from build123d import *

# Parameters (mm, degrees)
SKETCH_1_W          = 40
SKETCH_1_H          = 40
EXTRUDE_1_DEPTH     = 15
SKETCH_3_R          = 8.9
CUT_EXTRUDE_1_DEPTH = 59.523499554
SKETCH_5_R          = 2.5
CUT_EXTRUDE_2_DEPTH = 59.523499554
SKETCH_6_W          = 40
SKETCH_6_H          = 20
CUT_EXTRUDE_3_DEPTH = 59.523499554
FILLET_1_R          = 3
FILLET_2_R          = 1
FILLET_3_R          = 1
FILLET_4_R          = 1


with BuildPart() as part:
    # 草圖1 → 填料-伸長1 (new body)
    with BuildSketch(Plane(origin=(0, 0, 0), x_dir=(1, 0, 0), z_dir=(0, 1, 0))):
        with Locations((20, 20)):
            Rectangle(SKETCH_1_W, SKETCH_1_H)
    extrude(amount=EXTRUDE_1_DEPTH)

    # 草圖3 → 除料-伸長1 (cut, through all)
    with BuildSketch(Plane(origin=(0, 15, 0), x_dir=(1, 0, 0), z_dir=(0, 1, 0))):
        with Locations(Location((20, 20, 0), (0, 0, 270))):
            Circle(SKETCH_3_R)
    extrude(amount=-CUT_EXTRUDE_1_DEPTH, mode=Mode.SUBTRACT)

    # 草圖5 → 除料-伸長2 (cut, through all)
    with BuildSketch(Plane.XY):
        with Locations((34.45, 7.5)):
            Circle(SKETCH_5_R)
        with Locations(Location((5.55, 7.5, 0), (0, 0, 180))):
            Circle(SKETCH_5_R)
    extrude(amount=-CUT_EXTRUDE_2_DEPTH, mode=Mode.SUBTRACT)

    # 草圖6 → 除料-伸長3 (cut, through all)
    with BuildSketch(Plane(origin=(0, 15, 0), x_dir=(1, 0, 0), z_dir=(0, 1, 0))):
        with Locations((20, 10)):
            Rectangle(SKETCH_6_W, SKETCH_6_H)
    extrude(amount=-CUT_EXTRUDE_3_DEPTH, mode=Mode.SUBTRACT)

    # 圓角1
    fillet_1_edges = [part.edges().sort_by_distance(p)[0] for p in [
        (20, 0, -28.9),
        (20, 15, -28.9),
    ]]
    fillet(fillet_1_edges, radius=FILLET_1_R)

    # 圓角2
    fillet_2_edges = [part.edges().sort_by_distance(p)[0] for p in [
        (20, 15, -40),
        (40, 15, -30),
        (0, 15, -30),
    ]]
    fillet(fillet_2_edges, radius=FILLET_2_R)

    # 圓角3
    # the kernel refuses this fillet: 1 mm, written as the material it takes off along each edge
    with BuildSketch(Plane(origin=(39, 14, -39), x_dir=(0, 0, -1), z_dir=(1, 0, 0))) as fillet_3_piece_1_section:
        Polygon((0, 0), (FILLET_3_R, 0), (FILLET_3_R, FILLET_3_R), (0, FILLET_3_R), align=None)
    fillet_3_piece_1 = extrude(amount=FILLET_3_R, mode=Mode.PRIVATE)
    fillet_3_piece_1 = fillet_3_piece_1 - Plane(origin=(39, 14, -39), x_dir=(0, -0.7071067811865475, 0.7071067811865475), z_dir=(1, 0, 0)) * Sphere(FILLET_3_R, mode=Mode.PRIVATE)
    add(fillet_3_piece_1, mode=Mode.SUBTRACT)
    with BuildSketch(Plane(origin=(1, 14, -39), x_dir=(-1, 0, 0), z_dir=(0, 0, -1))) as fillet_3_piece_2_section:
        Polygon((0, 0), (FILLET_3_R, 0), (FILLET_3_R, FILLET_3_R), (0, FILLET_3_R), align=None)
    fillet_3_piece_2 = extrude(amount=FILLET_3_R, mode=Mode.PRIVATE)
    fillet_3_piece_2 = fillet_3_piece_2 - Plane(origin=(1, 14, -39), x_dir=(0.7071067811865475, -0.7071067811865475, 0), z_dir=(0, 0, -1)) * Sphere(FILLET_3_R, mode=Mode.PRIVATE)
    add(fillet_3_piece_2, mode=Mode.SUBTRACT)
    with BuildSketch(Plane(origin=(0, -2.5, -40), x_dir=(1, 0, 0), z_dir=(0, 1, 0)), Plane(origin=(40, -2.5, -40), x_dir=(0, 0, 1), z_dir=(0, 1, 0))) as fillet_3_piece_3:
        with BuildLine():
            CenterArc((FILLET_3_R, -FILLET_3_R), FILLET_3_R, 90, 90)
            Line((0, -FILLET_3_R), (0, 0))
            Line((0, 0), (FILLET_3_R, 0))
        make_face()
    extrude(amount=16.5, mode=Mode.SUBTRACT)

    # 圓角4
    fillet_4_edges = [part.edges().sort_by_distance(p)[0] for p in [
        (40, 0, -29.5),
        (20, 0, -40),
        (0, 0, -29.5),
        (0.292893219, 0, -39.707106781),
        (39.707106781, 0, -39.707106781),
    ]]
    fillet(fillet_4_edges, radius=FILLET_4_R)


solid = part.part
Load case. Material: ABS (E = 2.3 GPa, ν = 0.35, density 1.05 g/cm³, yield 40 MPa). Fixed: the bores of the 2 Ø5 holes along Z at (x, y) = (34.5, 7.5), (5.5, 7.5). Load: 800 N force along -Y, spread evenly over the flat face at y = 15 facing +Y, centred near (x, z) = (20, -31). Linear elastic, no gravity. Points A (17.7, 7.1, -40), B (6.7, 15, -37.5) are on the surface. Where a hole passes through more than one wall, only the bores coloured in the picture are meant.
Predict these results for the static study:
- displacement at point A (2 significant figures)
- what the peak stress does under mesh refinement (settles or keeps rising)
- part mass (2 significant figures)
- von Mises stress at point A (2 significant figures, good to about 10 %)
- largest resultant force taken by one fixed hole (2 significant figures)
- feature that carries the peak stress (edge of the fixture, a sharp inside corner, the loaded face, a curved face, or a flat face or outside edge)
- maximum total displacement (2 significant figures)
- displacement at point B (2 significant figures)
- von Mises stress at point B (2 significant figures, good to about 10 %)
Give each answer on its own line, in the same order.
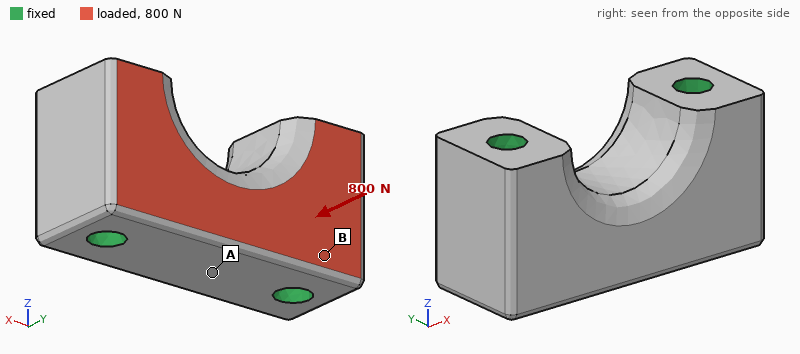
15 µm
keeps rising
9.7 g
0.77 MPa
400 N
edge of the fixture
17 µm
5.7 µm
2.0 MPa
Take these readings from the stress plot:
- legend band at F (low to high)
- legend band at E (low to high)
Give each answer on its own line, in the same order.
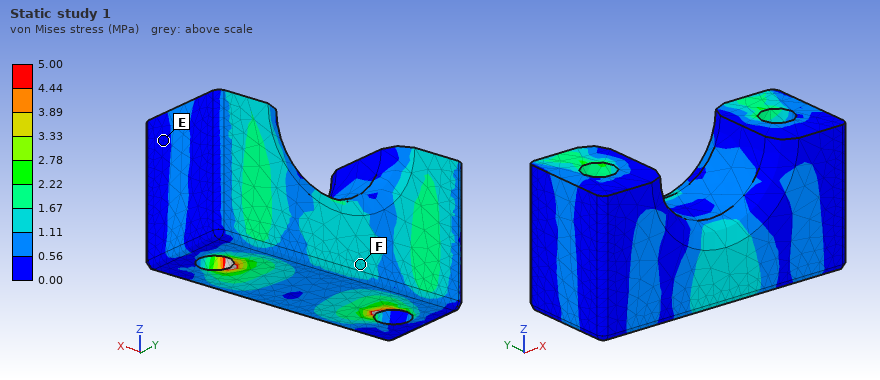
1.11 to 1.67 MPa
0.00 to 0.56 MPa
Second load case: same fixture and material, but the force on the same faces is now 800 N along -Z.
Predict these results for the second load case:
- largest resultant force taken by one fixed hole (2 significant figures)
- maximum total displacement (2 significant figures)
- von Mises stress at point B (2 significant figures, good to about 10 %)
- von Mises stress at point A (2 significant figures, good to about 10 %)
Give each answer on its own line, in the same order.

400 N
33 µm
3.2 MPa
1.4 MPa
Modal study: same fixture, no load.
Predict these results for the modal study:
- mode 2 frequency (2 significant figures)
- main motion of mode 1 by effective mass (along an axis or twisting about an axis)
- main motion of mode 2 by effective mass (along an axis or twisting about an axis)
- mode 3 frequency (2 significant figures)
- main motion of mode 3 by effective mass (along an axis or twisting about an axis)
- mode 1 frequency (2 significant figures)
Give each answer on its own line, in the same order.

16 kHz
along Y
along Z
19 kHz
twisting about X
13 kHz
